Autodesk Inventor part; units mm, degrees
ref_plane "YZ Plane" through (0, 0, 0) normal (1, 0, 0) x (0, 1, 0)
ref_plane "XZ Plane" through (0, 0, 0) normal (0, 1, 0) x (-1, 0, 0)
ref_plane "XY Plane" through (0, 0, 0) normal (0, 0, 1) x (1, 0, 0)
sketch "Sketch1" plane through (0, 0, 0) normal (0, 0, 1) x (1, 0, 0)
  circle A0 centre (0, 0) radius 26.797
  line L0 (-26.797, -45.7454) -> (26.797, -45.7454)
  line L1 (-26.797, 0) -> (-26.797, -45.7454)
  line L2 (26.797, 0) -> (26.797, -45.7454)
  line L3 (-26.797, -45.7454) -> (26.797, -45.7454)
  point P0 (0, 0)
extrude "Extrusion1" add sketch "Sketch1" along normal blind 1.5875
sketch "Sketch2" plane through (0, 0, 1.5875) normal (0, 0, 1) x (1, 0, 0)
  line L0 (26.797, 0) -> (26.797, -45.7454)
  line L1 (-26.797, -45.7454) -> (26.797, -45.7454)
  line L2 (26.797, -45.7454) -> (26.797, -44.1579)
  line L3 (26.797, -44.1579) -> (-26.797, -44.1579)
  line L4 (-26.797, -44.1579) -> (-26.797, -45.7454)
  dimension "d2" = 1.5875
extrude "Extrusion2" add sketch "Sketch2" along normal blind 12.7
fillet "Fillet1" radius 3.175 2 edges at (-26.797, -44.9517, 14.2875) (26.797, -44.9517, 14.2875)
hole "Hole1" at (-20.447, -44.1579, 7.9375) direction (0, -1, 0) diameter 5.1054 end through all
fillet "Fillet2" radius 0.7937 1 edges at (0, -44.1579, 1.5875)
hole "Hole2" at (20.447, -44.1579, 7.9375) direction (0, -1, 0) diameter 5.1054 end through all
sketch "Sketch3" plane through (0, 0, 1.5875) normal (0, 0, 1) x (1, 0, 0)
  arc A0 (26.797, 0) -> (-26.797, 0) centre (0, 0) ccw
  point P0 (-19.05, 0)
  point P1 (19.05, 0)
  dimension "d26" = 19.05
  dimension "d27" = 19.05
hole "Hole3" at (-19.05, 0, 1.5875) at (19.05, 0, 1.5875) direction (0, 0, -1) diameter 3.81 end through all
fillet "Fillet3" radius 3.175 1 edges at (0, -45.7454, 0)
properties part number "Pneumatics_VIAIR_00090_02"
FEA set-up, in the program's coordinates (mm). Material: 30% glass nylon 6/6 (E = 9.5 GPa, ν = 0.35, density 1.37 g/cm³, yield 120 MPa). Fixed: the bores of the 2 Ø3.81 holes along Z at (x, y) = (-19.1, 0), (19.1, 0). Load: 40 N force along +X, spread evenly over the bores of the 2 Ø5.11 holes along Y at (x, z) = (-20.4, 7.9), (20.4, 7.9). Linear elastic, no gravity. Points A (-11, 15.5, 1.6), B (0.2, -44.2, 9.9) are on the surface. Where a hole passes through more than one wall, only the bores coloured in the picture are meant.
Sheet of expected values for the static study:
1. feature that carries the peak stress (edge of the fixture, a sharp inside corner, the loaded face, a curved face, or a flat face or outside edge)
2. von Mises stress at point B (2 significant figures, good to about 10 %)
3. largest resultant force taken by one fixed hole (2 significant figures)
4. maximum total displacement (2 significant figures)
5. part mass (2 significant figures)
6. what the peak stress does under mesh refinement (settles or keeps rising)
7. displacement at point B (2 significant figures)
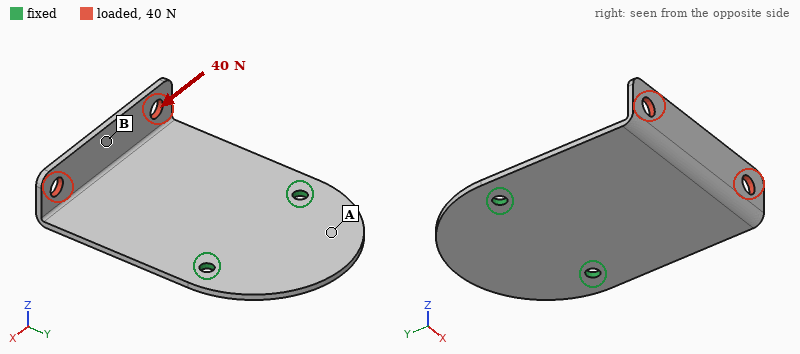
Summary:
edge of the fixture
5.5 MPa
50 N
0.93 mm
9.0 g
keeps rising
0.30 mm
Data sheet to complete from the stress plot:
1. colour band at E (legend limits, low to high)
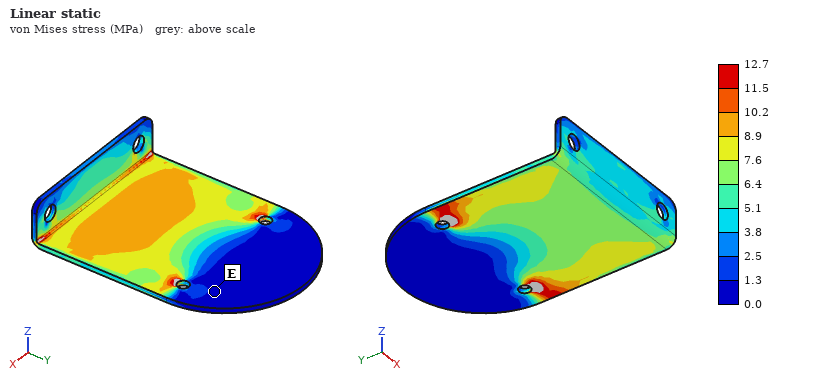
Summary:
0.0 to 1.3 MPa
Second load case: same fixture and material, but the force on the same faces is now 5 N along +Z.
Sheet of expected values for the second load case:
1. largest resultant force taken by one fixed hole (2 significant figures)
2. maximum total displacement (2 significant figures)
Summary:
2.5 N
1.00 mm
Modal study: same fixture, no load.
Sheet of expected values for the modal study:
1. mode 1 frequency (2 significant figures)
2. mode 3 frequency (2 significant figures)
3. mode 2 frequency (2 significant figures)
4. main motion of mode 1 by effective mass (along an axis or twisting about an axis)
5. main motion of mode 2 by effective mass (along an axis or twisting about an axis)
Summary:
230 Hz
1100 Hz
550 Hz
along Z
twisting about Y
